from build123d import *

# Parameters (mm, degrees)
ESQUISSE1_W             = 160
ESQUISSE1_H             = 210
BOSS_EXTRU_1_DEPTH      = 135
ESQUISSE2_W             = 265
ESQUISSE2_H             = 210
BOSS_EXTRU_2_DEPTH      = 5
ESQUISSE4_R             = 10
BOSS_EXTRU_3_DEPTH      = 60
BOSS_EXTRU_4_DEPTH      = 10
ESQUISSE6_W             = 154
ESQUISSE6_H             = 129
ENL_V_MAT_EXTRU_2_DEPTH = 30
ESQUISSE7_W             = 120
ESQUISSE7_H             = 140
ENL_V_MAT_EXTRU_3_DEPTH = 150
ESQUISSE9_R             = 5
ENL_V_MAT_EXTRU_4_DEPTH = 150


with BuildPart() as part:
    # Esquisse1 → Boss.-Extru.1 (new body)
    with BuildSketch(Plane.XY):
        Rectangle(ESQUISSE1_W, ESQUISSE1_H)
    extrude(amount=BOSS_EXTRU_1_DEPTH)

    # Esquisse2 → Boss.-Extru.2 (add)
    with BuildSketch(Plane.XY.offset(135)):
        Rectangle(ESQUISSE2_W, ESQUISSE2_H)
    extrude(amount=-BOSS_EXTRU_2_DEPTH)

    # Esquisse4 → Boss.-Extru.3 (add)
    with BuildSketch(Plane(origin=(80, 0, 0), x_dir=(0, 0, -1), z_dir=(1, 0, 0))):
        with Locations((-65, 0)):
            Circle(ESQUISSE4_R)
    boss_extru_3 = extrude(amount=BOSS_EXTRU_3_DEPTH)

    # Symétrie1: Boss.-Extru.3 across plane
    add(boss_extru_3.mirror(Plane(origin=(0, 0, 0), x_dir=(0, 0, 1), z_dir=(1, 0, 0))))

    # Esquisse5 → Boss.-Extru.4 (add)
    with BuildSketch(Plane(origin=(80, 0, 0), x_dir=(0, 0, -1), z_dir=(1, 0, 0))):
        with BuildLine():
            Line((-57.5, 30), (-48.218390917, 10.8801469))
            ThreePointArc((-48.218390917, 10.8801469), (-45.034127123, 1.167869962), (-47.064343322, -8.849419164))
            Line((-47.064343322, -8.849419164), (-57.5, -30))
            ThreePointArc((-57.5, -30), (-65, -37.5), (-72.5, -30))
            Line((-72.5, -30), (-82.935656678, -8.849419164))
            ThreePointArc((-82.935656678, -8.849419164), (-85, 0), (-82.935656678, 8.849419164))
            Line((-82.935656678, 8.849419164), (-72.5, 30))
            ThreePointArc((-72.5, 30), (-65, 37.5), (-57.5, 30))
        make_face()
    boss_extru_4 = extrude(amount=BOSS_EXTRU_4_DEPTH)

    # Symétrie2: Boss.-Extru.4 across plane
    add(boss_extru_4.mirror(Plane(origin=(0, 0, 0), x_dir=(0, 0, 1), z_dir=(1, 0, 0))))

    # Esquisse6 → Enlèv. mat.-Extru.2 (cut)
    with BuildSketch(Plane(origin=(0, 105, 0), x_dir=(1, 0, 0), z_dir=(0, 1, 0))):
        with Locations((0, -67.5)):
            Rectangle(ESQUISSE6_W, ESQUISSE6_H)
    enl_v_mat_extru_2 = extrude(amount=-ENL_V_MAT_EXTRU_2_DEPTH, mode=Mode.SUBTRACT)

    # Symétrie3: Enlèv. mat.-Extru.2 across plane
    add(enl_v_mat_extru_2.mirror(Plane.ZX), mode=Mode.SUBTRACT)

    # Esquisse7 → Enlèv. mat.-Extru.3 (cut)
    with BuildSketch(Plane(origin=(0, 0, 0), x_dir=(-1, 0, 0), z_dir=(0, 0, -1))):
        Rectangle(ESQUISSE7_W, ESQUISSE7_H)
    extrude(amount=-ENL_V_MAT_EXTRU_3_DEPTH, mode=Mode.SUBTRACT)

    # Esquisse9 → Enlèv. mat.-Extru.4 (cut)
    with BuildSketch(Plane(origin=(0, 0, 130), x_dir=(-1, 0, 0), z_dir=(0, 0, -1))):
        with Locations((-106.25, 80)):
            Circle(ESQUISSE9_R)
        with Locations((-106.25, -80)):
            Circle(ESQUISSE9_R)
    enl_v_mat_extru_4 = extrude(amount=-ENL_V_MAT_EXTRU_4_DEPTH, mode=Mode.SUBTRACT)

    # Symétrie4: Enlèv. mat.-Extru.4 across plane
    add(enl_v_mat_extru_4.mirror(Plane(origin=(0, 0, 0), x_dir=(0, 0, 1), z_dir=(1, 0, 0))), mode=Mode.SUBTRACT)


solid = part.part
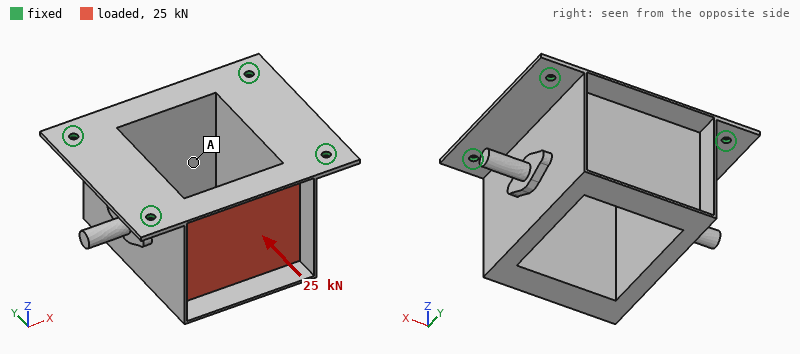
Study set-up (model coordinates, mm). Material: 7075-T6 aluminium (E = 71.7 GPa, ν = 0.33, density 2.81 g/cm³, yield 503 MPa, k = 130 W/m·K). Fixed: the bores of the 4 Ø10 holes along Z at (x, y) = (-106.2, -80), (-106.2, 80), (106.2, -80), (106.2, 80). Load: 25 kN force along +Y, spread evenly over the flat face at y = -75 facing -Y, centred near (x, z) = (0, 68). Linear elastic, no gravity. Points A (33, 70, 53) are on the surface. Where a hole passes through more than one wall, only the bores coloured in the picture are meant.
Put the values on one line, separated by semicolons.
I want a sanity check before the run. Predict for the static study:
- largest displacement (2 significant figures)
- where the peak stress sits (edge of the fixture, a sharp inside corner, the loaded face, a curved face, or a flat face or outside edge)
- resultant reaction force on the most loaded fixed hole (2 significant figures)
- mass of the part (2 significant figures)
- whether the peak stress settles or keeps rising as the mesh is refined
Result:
1.1 mm; edge of the fixture; 9.3 kN; 3.5 kg; keeps rising
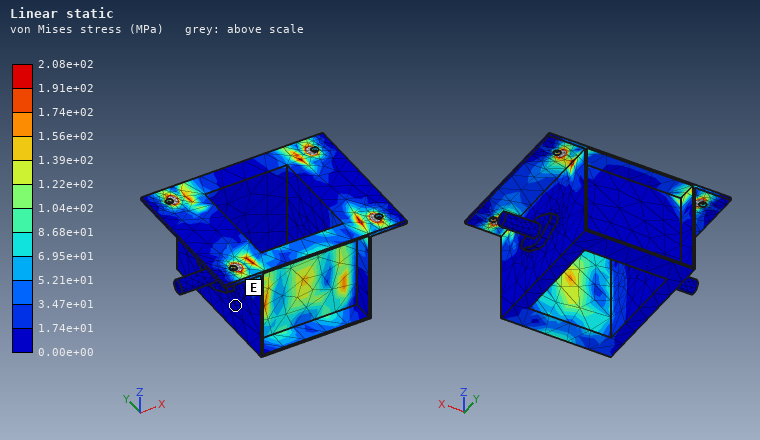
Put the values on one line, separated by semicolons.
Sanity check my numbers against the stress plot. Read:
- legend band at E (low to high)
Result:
0.00e+00 to 1.74e+01 MPa
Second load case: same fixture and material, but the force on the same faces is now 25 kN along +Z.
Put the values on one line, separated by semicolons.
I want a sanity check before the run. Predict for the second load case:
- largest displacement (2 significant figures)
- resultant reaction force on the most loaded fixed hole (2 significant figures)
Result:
1.1 mm; 13 kN
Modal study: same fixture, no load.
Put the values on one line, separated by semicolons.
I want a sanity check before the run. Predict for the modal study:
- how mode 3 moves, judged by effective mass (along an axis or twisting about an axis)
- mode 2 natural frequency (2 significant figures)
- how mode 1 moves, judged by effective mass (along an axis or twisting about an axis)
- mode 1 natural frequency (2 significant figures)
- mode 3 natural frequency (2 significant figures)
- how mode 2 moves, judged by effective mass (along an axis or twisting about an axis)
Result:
along Z; 640 Hz; along Y; 600 Hz; 710 Hz; along X
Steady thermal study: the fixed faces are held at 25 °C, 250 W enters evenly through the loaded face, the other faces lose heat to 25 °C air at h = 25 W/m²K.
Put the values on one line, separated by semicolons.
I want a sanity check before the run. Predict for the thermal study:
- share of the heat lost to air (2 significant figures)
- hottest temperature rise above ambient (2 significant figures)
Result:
64 %; 65 K
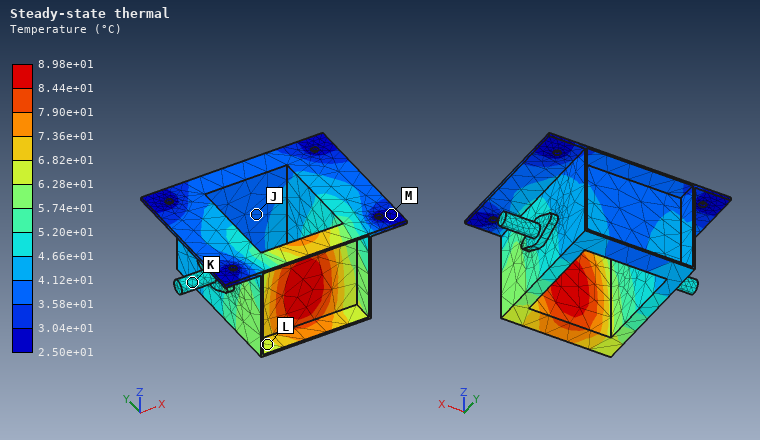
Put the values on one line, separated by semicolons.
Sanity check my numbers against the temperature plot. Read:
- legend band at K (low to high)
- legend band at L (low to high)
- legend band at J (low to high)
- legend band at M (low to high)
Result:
4.66e+01 to 5.20e+01 °C; 6.28e+01 to 6.82e+01 °C; 3.58e+01 to 4.12e+01 °C; 2.50e+01 to 3.04e+01 °C
